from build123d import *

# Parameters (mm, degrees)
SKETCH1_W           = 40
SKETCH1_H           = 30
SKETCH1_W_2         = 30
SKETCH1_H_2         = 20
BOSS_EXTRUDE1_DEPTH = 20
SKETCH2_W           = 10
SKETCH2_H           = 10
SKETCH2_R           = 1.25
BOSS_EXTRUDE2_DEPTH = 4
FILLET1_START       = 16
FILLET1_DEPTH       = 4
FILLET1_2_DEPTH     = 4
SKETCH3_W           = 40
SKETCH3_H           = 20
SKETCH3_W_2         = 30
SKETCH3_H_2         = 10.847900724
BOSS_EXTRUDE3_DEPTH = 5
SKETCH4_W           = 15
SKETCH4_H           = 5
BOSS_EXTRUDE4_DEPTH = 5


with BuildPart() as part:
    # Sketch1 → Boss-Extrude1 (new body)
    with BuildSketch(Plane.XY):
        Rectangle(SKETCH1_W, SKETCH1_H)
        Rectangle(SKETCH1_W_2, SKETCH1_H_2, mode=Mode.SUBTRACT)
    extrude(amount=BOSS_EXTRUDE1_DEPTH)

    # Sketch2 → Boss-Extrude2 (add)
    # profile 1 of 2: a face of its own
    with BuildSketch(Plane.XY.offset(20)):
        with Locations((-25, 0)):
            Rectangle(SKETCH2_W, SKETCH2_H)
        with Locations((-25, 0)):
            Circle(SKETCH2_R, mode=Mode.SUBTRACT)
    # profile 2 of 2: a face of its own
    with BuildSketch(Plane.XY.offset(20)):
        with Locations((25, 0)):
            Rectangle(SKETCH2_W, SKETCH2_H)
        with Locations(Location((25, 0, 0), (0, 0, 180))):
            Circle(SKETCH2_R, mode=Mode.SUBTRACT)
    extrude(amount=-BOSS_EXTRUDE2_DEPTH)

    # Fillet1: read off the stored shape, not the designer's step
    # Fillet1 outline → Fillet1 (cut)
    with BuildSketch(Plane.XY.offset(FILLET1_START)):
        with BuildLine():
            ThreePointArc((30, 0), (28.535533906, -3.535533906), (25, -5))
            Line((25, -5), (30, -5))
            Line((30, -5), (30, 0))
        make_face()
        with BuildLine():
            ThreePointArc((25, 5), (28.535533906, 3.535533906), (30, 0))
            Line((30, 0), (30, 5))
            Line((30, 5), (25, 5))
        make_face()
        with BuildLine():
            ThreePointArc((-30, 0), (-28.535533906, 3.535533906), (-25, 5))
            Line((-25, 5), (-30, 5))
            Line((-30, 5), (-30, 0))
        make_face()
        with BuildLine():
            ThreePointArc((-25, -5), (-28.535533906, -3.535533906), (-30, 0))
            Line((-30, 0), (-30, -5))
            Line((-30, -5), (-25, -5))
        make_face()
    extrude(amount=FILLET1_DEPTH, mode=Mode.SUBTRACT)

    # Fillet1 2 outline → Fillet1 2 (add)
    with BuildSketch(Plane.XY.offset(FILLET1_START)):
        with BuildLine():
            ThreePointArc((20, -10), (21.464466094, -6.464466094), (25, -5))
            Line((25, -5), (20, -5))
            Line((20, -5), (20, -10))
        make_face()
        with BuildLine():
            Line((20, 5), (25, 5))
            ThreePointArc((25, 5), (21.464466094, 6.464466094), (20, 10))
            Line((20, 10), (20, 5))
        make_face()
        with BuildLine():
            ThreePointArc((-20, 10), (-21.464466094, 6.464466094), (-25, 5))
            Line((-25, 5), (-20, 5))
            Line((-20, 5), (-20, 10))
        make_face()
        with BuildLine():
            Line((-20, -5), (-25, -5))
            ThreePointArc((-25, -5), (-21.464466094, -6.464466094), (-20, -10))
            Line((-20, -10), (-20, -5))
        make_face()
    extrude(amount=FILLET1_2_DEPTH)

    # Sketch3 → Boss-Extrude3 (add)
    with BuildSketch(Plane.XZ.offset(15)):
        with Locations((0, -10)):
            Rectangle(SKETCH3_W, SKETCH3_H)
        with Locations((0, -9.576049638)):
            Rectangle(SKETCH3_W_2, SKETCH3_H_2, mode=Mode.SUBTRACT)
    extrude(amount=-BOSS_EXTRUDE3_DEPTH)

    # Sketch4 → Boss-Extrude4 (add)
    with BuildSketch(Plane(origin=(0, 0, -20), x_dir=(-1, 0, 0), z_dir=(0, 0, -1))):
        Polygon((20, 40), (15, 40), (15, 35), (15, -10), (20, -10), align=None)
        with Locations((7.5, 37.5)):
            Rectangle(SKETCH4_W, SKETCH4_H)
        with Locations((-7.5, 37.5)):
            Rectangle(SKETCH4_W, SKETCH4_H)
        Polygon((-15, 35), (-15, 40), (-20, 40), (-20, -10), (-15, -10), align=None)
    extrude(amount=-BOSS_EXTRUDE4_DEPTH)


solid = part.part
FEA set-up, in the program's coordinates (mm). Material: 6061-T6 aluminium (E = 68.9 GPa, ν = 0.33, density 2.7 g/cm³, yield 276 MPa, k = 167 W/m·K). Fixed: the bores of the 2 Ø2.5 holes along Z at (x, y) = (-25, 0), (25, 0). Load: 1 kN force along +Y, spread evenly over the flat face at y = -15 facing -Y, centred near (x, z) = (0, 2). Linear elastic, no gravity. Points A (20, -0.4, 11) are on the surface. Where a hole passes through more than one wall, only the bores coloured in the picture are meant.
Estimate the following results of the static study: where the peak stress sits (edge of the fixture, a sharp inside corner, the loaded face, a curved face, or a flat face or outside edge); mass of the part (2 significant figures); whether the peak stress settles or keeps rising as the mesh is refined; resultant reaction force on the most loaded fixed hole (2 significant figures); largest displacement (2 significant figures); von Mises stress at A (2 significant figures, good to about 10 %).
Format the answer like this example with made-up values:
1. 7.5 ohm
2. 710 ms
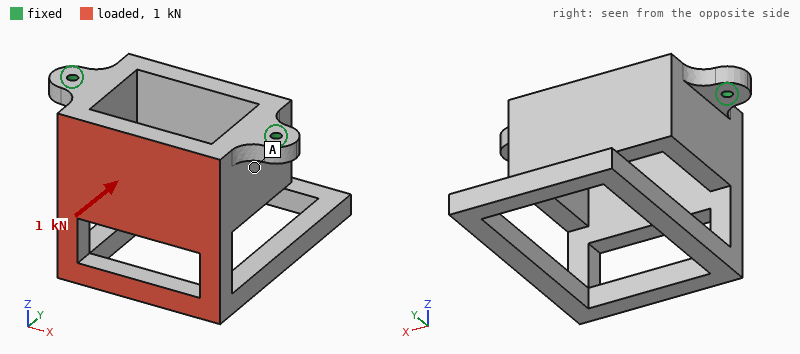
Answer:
1. edge of the fixture
2. 50 g
3. keeps rising
4. 510 N
5. 0.70 mm
6. 26 MPa
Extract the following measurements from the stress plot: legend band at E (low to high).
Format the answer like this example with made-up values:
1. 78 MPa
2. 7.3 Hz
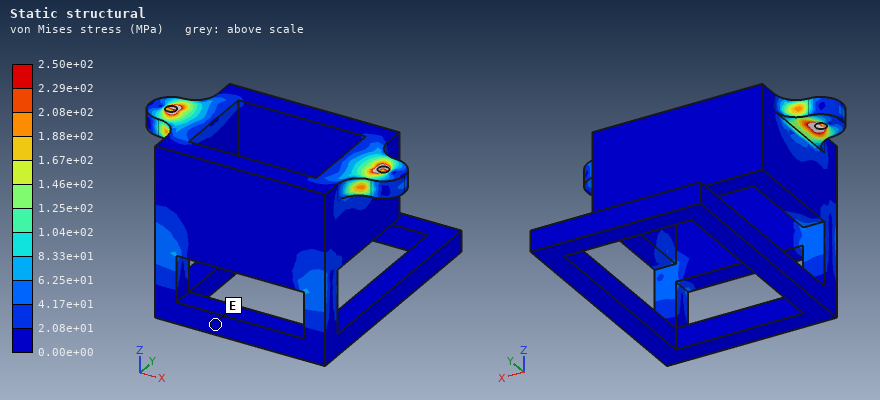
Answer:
1. 0.00e+00 to 2.08e+01 MPa
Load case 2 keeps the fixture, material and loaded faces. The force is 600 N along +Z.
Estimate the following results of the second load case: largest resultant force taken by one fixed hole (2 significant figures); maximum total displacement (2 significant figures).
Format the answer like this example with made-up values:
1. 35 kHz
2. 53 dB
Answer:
1. 320 N
2. 0.30 mm
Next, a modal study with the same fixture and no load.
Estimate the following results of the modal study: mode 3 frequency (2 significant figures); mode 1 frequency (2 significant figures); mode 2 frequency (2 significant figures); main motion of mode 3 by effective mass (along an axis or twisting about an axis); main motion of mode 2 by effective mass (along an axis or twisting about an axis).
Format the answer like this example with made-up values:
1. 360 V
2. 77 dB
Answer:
1. 1500 Hz
2. 660 Hz
3. 1100 Hz
4. along Y
5. along X
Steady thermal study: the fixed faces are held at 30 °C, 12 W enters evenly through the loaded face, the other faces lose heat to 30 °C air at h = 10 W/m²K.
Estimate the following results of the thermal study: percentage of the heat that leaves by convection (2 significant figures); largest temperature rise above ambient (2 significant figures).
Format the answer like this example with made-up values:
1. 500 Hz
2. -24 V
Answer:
1. 7.1 %
2. 16 K
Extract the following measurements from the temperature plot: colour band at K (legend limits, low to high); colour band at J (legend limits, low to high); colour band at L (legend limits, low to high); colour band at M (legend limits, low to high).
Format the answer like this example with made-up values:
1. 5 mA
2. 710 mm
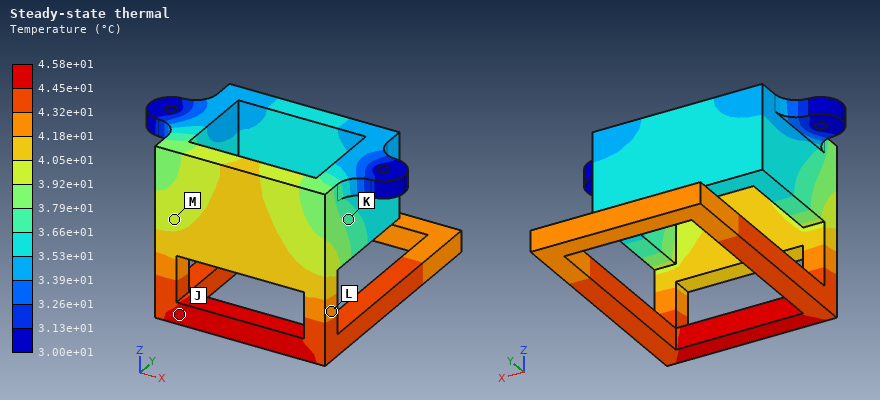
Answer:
1. 3.66e+01 to 3.79e+01 °C
2. 4.45e+01 to 4.58e+01 °C
3. 4.18e+01 to 4.32e+01 °C
4. 3.92e+01 to 4.05e+01 °C
